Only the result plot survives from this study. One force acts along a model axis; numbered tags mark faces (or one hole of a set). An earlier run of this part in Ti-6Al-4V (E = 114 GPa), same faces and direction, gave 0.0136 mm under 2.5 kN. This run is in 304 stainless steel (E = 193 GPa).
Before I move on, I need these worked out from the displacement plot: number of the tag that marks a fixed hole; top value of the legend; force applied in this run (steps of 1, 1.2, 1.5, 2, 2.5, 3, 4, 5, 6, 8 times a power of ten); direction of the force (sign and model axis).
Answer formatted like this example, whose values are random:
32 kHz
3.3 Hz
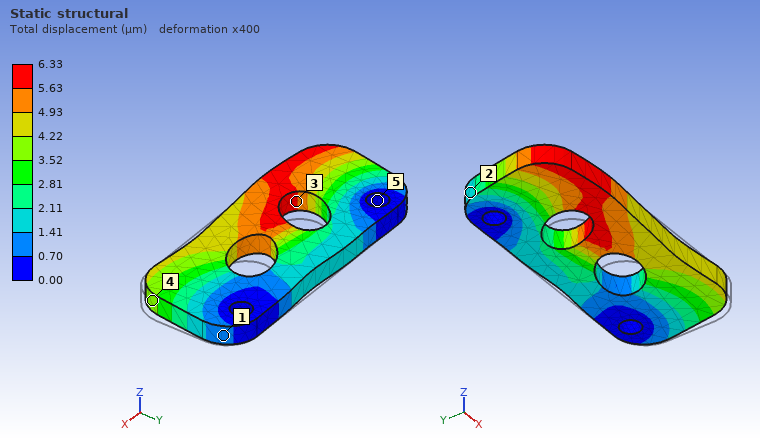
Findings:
5
6.33 µm
2 kN
-X
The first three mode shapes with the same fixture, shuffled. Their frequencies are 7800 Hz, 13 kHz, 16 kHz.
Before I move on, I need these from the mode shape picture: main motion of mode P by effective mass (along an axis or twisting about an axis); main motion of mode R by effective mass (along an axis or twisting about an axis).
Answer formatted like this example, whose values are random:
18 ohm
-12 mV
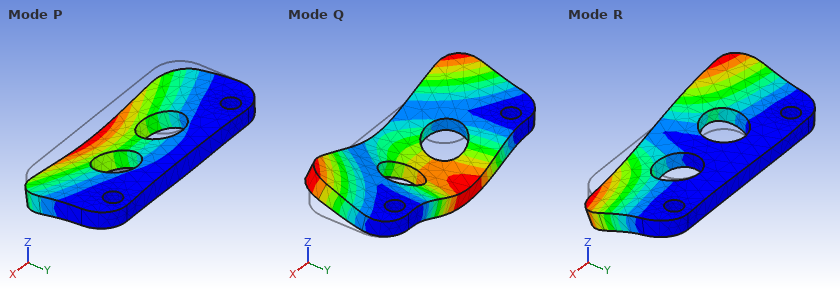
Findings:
along Z
twisting about Y
